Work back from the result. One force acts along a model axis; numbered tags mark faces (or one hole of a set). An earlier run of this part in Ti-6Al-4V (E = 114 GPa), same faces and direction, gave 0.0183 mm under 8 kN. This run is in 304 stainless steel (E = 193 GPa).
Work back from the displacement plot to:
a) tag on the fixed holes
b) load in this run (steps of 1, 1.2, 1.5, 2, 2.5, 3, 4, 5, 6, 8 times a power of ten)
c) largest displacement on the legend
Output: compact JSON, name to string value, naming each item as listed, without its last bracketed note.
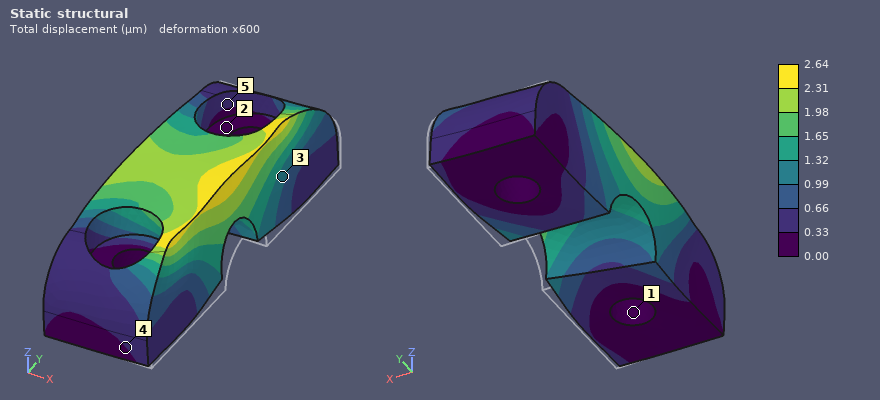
{"tag on the fixed holes": "1", "load in this run": "2 kN", "largest displacement on the legend": "2.64 µm"}
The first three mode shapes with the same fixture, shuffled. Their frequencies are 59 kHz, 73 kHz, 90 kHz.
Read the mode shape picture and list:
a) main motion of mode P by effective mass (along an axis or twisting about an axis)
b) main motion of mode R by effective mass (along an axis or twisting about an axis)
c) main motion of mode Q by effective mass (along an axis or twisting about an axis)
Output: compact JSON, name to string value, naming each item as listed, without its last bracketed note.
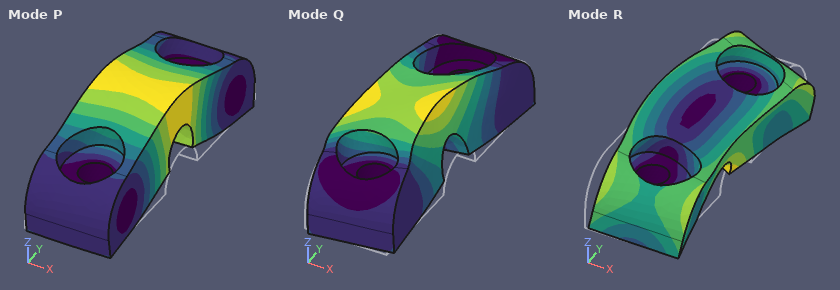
{"main motion of mode P by effective mass": "along Z", "main motion of mode R by effective mass": "twisting about Y", "main motion of mode Q by effective mass": "along X"}
